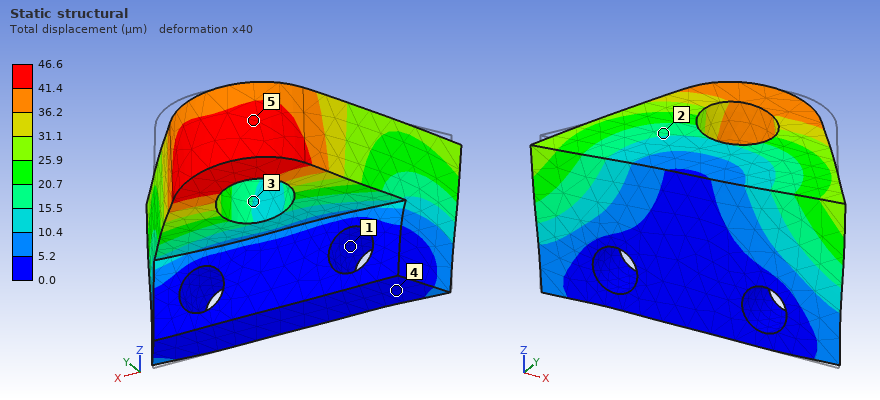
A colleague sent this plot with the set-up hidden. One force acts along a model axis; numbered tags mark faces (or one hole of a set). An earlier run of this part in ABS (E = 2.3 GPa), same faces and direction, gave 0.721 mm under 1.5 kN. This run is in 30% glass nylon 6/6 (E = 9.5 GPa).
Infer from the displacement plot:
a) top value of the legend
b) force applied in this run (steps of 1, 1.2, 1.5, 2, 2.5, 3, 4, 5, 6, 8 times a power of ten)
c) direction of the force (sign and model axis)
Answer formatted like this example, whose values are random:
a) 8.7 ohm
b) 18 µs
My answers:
a) 46.6 µm
b) 400 N
c) -X
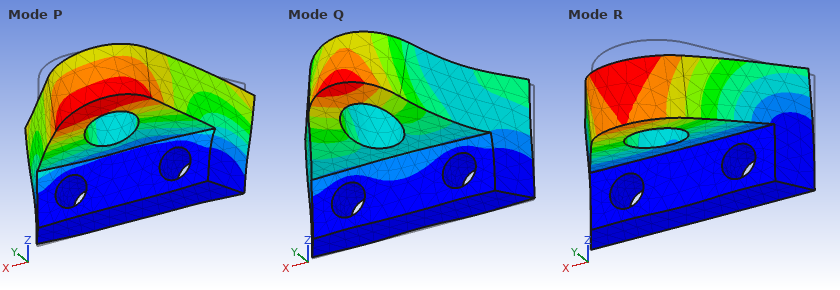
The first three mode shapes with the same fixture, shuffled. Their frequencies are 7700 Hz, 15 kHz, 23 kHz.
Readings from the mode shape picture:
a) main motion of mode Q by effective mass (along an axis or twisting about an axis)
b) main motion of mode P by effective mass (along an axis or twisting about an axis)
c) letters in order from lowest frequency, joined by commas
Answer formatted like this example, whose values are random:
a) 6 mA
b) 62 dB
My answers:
a) along Y
b) along X
c) R, P, Q
